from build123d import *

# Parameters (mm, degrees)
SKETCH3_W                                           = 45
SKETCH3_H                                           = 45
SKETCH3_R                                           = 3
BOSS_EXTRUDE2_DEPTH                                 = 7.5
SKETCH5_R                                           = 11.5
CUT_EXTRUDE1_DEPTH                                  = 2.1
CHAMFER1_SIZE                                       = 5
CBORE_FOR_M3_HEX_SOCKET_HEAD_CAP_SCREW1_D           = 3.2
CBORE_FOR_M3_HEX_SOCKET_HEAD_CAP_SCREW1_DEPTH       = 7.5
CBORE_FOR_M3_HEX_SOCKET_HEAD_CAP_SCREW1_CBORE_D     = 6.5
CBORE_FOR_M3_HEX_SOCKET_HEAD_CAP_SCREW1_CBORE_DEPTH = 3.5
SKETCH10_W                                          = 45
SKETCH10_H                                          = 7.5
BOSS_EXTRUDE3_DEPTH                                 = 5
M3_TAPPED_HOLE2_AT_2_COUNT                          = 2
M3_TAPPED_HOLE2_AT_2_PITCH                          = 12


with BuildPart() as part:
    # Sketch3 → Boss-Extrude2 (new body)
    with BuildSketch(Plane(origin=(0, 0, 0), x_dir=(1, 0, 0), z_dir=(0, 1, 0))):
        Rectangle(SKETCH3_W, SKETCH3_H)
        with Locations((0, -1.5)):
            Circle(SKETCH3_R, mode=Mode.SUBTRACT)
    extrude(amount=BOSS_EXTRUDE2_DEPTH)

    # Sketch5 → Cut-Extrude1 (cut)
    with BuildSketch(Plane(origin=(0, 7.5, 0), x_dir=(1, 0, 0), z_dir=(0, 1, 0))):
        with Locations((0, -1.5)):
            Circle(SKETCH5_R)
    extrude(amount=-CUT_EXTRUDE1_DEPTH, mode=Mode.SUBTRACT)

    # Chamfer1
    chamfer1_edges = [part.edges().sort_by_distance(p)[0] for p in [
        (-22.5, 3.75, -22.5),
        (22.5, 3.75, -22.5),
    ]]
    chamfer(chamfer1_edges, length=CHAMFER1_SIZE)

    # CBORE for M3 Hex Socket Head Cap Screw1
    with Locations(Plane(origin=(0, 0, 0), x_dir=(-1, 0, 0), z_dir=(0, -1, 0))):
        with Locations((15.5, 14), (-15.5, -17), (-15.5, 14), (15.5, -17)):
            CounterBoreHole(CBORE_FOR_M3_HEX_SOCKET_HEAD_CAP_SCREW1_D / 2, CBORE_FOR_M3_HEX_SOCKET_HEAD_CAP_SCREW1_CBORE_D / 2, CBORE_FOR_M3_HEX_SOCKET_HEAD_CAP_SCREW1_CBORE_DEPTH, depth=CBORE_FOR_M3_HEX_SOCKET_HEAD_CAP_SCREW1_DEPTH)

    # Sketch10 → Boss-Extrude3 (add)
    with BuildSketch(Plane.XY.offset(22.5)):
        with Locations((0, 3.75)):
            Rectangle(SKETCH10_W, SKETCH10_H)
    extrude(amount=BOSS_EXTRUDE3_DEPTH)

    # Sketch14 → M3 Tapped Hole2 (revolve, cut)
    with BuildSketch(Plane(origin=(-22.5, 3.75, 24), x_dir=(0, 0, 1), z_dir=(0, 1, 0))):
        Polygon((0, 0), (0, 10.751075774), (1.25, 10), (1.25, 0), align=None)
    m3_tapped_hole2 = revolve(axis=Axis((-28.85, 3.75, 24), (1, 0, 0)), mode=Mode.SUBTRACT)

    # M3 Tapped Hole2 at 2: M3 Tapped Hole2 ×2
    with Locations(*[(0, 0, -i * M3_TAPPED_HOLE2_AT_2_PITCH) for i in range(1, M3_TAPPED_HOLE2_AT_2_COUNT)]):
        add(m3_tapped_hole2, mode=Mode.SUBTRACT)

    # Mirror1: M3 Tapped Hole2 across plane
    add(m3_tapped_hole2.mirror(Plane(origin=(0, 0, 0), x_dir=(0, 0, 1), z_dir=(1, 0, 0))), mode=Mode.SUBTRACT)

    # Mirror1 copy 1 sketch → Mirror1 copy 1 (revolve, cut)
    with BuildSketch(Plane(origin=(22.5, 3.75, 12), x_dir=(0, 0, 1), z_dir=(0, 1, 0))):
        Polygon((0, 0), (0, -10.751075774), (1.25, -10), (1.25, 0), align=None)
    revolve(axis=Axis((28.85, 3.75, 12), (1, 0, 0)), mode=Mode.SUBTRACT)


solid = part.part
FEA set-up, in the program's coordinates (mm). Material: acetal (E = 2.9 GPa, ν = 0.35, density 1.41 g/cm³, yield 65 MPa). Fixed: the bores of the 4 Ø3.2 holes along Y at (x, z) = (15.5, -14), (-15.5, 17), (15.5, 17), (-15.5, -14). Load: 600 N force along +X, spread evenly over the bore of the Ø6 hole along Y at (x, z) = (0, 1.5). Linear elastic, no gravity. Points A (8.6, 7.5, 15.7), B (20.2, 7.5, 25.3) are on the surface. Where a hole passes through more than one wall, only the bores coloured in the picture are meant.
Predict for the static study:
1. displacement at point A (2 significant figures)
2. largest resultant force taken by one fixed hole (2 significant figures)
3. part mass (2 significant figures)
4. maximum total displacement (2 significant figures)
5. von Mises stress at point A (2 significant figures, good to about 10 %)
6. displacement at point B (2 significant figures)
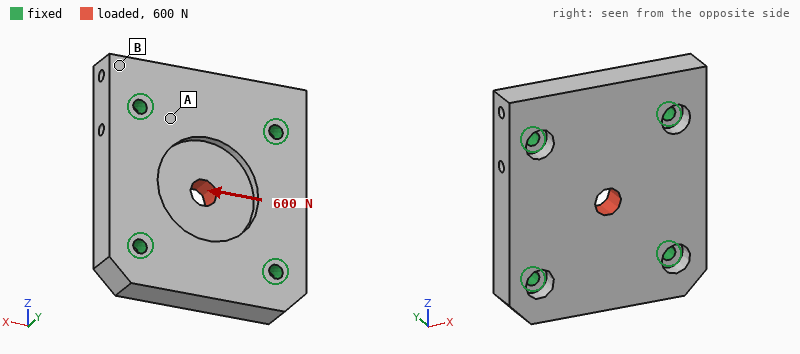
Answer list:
5.3 µm
160 N
21 g
30 µm
2.2 MPa
4.7 µm
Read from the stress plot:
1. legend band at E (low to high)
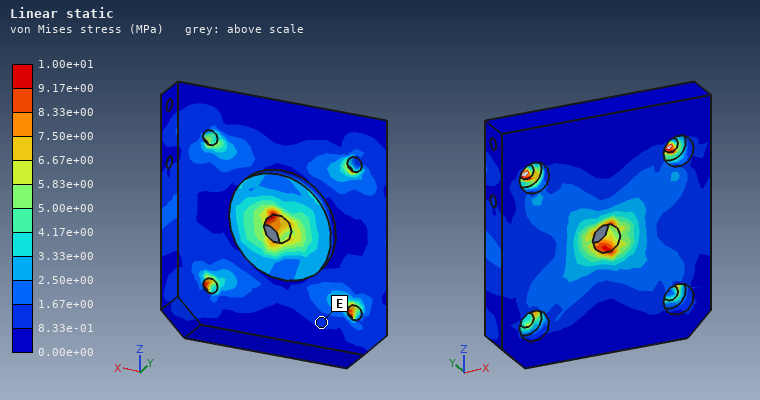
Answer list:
8.33e-01 to 1.67e+00 MPa
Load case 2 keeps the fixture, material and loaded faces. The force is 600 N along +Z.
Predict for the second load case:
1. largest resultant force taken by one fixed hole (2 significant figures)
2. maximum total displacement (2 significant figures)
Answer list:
160 N
29 µm
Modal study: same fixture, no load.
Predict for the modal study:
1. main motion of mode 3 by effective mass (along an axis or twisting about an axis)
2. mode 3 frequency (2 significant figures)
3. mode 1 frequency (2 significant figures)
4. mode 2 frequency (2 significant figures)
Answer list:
twisting about X
6200 Hz
5300 Hz
5400 Hz
